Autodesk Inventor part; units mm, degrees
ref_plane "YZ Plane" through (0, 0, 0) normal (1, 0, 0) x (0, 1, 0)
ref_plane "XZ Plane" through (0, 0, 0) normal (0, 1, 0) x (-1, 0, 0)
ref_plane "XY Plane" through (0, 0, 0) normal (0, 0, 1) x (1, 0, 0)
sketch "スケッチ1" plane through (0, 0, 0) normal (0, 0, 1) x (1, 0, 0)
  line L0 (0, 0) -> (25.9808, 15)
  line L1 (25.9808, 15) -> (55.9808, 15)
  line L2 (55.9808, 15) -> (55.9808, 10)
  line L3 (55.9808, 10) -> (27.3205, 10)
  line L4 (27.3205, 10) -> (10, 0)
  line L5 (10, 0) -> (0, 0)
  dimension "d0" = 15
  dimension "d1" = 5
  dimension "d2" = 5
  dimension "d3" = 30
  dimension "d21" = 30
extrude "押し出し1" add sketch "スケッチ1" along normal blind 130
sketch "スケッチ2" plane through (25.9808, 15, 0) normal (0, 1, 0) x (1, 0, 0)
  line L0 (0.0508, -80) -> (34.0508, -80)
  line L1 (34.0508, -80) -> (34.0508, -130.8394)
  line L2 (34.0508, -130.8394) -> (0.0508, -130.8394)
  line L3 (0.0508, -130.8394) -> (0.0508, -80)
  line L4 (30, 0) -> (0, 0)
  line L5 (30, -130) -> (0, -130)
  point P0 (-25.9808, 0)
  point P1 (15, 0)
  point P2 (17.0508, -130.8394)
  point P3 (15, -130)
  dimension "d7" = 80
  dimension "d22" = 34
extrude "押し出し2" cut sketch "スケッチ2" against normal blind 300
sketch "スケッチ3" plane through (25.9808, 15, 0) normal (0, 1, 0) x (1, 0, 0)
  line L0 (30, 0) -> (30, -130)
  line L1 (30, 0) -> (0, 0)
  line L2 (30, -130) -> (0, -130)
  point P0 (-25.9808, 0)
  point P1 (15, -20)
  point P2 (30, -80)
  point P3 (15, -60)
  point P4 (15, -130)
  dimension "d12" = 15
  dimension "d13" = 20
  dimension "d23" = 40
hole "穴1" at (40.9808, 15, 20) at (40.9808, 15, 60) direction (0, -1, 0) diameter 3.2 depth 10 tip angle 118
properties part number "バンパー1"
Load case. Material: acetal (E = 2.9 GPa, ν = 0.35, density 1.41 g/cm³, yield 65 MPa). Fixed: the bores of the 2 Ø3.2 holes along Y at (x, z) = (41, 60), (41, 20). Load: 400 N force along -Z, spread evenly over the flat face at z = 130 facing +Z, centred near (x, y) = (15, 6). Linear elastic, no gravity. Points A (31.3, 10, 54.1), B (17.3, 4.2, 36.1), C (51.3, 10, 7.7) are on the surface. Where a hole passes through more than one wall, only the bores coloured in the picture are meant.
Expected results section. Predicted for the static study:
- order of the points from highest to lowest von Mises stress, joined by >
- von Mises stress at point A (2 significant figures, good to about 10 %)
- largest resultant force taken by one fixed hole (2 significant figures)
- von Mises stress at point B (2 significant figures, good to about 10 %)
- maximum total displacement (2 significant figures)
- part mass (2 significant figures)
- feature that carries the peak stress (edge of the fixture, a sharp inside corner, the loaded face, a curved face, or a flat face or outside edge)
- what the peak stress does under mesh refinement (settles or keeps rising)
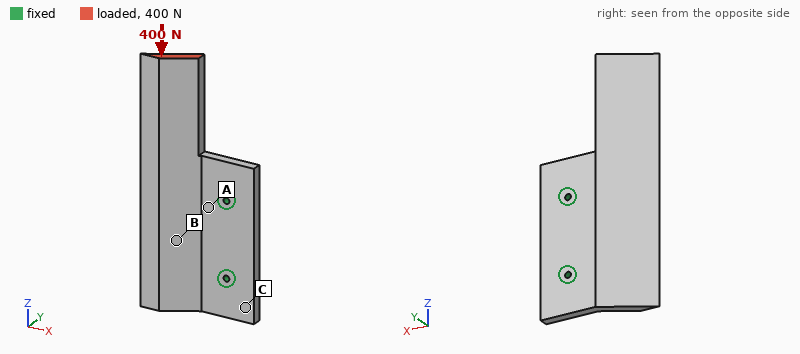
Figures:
A > B > C
5.2 MPa
330 N
3.0 MPa
0.49 mm
39 g
edge of the fixture
keeps rising
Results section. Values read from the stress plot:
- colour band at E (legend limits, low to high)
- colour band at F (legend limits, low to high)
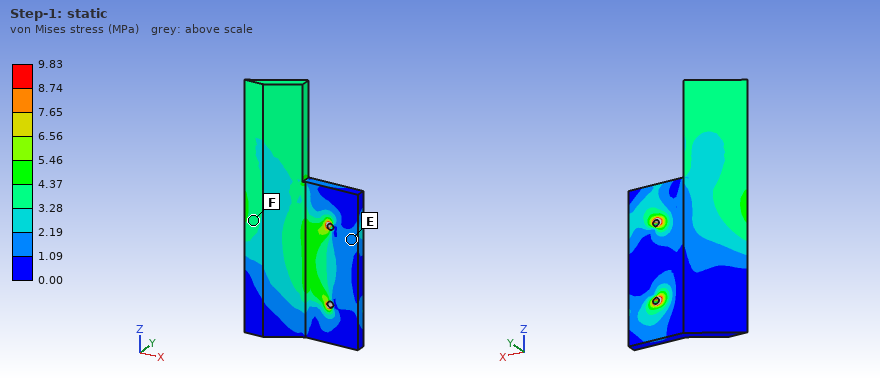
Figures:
1.09 to 2.19 MPa
3.28 to 4.37 MPa
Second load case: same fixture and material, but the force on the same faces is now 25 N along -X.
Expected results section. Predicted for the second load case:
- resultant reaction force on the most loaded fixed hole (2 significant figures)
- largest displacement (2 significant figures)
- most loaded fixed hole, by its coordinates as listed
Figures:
68 N
1.7 mm
(41, 60)
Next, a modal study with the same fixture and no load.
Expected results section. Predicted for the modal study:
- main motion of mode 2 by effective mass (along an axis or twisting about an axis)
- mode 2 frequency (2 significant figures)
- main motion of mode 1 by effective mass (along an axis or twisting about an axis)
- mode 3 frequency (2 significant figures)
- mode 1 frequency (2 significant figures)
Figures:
along Y
580 Hz
along Y
800 Hz
230 Hz
